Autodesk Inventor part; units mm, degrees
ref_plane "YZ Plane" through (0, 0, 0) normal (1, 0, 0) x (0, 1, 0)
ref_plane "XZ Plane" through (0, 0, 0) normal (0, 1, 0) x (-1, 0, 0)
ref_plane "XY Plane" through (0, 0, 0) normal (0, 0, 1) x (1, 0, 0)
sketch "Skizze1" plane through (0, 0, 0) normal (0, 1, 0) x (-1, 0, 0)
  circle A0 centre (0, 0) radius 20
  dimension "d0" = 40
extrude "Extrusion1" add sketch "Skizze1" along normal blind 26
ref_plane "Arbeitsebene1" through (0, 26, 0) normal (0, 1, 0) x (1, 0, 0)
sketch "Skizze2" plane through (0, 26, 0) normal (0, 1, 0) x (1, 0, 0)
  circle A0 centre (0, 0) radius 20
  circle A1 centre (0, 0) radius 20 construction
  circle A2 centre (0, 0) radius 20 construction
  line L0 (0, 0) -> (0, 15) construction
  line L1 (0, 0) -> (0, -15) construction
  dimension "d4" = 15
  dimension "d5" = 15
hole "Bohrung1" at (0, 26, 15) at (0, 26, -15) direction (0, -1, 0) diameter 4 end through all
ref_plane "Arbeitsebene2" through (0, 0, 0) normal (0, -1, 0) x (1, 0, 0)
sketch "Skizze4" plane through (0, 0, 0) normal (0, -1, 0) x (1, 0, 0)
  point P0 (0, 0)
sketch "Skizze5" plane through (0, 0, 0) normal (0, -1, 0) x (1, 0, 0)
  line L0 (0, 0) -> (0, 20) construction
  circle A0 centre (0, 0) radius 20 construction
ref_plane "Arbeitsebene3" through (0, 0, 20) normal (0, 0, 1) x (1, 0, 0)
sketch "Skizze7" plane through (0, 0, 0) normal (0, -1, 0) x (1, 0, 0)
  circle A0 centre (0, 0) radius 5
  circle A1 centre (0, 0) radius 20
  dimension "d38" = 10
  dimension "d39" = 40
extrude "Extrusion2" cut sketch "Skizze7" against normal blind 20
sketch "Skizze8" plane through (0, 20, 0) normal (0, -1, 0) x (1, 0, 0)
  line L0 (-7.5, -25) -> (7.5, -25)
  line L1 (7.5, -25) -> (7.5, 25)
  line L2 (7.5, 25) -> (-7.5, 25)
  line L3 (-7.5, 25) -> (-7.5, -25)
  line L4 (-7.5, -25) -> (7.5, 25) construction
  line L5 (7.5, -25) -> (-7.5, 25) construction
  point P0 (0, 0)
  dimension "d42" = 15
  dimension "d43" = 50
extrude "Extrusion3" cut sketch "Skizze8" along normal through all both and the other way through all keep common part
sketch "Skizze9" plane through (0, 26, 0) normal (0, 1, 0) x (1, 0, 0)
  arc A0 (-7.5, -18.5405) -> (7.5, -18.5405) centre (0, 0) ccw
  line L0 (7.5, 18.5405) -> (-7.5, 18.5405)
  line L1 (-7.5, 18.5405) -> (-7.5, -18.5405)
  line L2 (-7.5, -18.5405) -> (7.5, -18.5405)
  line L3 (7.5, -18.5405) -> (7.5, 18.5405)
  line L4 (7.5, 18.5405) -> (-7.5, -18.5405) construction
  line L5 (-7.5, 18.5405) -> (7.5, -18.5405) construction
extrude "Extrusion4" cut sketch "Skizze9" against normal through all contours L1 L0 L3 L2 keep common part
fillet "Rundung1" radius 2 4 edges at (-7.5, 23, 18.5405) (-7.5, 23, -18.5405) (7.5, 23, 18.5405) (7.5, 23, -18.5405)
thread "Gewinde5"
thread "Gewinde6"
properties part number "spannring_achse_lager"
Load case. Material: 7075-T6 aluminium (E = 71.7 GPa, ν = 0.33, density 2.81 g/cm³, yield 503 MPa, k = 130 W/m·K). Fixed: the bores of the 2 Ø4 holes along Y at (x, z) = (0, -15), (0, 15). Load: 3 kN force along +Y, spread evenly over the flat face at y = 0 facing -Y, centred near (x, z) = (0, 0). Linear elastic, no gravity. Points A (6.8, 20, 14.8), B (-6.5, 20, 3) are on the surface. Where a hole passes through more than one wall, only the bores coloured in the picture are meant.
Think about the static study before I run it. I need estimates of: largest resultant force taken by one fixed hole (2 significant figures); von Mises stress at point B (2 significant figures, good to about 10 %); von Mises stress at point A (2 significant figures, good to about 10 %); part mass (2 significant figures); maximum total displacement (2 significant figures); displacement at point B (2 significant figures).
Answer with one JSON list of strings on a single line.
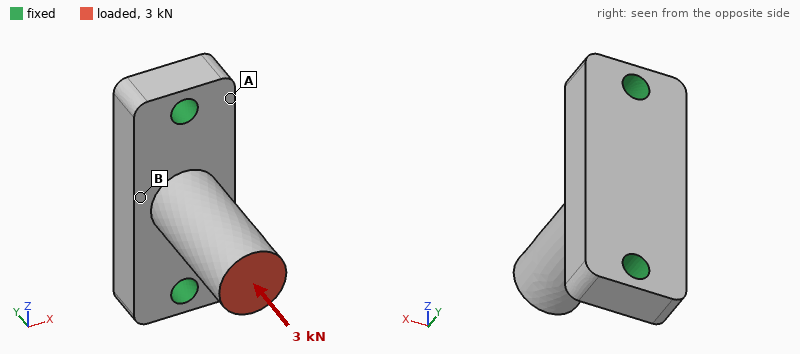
["1.5 kN", "55 MPa", "21 MPa", "13 g", "34 µm", "22 µm"]
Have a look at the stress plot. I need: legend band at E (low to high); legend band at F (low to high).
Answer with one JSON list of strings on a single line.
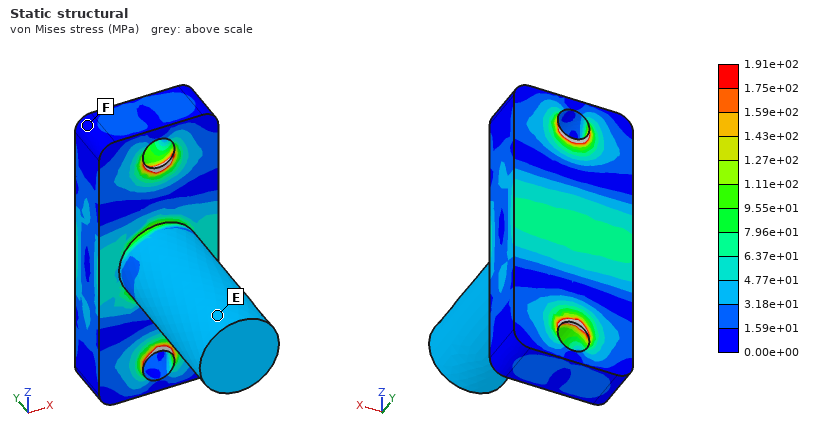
["3.18e+01 to 4.77e+01 MPa", "0.00e+00 to 1.59e+01 MPa"]
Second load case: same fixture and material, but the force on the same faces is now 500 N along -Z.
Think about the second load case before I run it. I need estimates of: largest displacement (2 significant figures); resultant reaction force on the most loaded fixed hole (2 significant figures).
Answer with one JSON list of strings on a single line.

["72 µm", "580 N"]
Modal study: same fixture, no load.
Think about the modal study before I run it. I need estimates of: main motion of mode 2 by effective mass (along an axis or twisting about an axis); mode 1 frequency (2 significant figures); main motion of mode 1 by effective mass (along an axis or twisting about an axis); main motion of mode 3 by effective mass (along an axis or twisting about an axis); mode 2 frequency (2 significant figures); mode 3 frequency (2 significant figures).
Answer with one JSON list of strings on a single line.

["along Z", "8100 Hz", "along X", "along Y", "12 kHz", "20 kHz"]
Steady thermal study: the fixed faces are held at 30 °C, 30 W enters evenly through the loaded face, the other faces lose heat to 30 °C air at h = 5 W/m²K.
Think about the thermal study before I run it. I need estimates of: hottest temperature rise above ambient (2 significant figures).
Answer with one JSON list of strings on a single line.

["78 K"]
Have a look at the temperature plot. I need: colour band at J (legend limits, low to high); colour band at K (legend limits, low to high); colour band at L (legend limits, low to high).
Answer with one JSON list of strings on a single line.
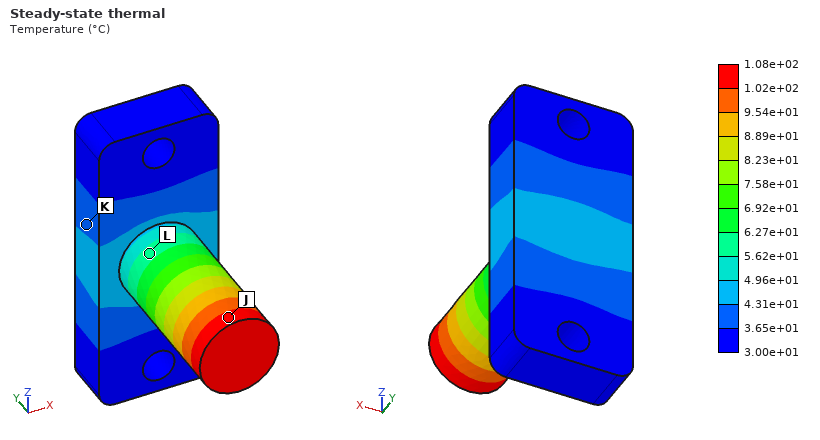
["1.02e+02 to 1.08e+02 °C", "3.65e+01 to 4.31e+01 °C", "5.62e+01 to 6.27e+01 °C"]
